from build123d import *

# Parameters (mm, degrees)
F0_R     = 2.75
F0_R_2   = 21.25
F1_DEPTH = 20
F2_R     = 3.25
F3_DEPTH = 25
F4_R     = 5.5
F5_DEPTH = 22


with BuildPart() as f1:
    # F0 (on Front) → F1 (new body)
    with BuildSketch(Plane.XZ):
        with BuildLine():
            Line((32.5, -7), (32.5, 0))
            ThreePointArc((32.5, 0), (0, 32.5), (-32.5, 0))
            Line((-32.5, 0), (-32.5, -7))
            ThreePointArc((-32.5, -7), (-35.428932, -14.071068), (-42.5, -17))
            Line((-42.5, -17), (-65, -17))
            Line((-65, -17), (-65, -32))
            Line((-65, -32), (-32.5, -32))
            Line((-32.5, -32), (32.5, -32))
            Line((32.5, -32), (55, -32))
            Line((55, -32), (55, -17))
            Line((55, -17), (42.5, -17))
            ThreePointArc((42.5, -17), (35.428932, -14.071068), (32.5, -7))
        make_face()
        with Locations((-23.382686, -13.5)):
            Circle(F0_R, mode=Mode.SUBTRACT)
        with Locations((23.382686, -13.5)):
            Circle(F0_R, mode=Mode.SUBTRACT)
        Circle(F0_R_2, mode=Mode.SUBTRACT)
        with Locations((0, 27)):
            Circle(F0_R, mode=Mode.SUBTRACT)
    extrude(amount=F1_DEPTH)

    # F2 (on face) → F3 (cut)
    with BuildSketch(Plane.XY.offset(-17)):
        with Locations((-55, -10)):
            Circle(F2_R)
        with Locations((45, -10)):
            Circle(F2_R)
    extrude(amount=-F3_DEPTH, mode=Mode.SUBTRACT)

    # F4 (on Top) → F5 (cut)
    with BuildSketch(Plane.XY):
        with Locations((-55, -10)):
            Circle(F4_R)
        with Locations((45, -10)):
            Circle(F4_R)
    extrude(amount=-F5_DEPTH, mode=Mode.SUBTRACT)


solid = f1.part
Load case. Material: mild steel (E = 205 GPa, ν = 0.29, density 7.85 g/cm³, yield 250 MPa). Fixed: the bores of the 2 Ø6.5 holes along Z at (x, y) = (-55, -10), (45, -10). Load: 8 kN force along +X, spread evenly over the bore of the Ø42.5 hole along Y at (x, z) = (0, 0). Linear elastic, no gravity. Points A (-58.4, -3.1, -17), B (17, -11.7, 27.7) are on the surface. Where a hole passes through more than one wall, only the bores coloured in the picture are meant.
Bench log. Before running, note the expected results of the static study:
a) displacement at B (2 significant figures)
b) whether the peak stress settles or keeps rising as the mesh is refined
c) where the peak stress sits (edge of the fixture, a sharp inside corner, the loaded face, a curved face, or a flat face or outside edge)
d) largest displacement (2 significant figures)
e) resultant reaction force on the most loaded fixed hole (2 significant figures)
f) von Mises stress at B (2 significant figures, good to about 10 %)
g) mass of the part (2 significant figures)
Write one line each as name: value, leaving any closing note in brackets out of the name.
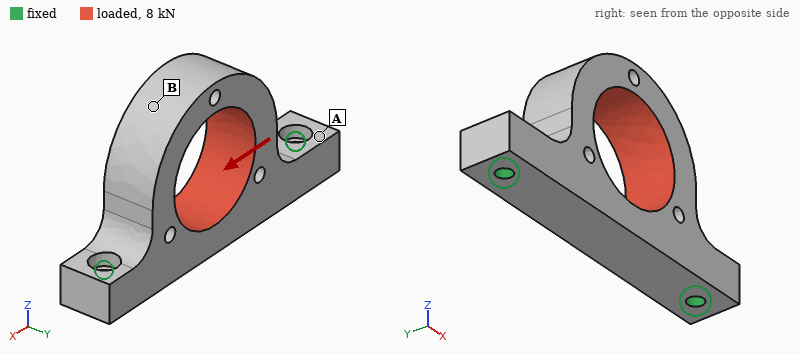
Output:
displacement at B: 22 µm
whether the peak stress settles or keeps rising as the mesh is refined: keeps rising
where the peak stress sits: edge of the fixture
largest displacement: 23 µm
resultant reaction force on the most loaded fixed hole: 4.6 kN
von Mises stress at B: 23 MPa
mass of the part: 480 g
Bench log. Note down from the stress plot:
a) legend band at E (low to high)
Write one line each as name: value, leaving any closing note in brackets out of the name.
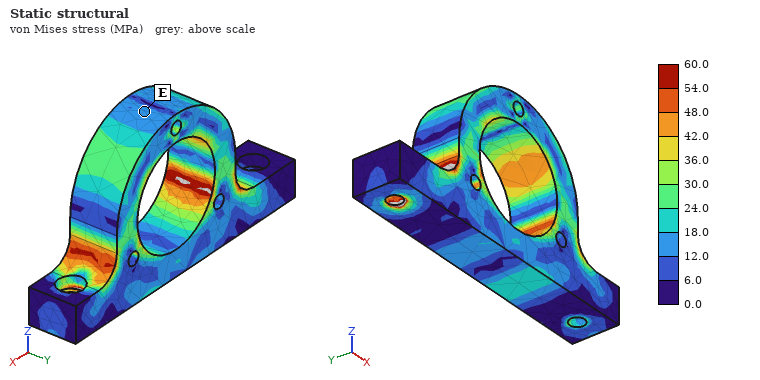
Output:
legend band at E: 12.0 to 18.0 MPa
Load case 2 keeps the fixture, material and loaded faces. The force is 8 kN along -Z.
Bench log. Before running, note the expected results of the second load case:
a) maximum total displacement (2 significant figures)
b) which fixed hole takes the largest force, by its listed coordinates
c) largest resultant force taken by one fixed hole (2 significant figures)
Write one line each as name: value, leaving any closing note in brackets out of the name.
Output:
maximum total displacement: 23 µm
which fixed hole takes the largest force, by its listed coordinates: (45, -10)
largest resultant force taken by one fixed hole: 4.7 kN
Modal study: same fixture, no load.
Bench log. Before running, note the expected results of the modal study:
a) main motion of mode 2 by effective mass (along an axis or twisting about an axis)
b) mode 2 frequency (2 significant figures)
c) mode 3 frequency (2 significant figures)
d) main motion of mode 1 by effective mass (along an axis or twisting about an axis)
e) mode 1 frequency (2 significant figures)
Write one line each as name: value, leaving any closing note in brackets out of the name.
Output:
main motion of mode 2 by effective mass: along Z
mode 2 frequency: 5500 Hz
mode 3 frequency: 6300 Hz
main motion of mode 1 by effective mass: along Y
mode 1 frequency: 2300 Hz
